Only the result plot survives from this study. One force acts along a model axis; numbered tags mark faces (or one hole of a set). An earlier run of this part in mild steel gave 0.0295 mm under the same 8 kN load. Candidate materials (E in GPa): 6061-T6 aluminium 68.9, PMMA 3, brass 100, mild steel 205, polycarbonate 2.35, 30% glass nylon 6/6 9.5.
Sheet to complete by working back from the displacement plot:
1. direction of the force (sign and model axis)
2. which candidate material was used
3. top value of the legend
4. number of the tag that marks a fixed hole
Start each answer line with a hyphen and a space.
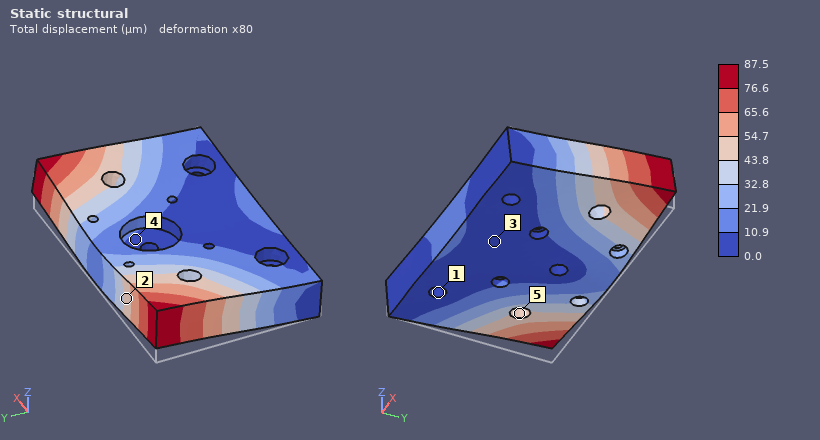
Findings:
- +Z
- 6061-T6 aluminium
- 87.5 µm
- 1
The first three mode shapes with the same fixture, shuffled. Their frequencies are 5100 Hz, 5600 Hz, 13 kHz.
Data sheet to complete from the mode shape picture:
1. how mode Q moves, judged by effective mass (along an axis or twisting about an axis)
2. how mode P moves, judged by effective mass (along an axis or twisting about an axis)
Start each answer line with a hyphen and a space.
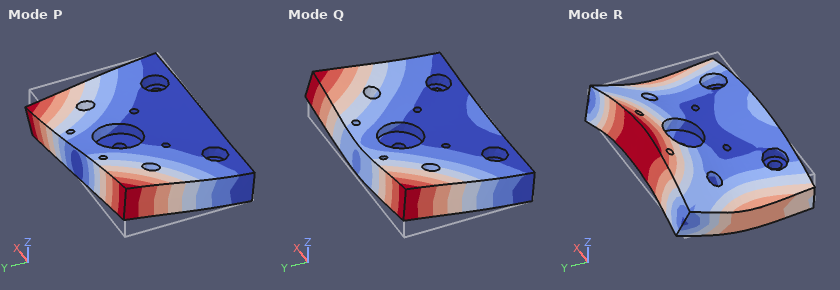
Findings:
- along Z
- twisting about Y
